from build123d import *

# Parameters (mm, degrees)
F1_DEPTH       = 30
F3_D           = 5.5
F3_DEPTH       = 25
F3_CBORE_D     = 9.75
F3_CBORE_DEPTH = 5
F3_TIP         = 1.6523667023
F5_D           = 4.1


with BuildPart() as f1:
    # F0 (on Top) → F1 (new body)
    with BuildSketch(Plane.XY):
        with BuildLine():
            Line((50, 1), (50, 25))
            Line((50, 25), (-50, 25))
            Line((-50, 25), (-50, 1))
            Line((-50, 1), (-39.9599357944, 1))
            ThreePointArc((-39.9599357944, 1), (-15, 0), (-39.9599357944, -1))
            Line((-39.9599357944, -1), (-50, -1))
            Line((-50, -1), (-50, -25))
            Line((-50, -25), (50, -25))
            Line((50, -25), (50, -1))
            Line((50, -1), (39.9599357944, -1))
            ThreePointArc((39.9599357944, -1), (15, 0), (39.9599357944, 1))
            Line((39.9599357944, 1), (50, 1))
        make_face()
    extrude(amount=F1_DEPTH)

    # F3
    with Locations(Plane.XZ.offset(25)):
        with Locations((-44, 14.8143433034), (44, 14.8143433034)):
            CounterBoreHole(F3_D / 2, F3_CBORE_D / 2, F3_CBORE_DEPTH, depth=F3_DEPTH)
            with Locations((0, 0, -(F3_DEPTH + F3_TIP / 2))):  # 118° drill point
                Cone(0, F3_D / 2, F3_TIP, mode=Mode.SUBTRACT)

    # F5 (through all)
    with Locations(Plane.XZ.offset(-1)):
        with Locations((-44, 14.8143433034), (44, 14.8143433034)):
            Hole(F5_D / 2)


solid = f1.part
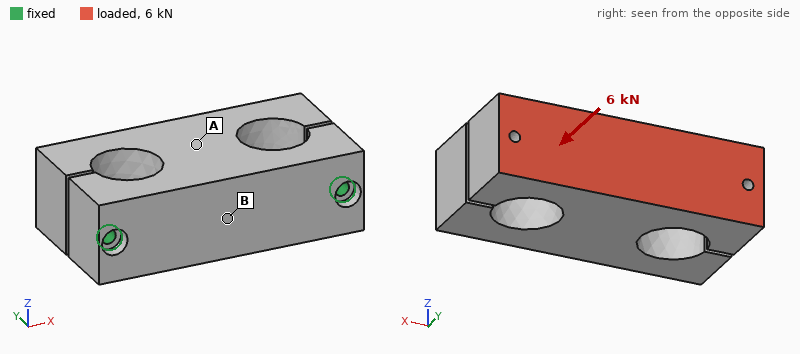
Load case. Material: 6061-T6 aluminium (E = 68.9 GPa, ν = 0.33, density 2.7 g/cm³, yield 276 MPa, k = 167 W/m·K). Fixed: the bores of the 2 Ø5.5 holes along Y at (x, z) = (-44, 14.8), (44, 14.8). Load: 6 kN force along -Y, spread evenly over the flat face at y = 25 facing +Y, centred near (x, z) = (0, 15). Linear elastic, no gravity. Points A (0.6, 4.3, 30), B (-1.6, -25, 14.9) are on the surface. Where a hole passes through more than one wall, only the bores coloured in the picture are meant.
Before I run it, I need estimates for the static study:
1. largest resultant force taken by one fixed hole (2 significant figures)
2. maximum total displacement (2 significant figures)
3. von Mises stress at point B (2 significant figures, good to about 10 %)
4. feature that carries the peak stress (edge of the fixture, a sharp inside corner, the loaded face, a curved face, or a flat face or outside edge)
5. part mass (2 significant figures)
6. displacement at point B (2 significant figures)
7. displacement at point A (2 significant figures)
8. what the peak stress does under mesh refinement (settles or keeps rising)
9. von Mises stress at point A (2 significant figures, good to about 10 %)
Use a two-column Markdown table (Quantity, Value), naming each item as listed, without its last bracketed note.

| Quantity | Value |
|---|---|
| largest resultant force taken by one fixed hole | 3.1 kN |
| maximum total displacement | 73 µm |
| von Mises stress at point B | 24 MPa |
| feature that carries the peak stress | edge of the fixture |
| part mass | 320 g |
| displacement at point B | 30 µm |
| displacement at point A | 31 µm |
| what the peak stress does under mesh refinement | keeps rising |
| von Mises stress at point A | 11 MPa |
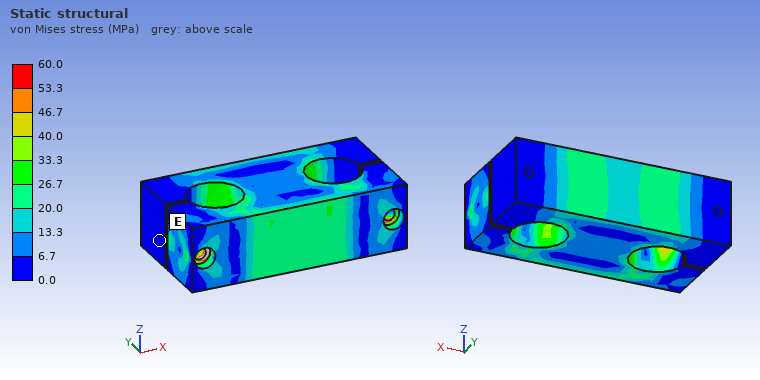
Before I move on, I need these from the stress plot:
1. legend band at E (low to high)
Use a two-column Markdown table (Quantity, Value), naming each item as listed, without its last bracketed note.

| Quantity | Value |
|---|---|
| legend band at E | 0.0 to 6.7 MPa |
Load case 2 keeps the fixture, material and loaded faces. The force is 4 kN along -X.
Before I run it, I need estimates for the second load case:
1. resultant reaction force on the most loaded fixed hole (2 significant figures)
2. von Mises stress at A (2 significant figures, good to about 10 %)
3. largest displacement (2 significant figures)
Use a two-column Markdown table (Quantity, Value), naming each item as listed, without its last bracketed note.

| Quantity | Value |
|---|---|
| resultant reaction force on the most loaded fixed hole | 3.2 kN |
| von Mises stress at A | 14 MPa |
| largest displacement | 98 µm |
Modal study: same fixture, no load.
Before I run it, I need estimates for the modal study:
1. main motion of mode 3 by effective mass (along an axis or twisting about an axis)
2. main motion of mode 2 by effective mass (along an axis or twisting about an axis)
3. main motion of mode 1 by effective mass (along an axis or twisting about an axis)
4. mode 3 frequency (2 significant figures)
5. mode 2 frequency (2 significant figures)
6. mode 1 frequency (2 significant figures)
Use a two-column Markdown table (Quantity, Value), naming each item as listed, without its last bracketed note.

| Quantity | Value |
|---|---|
| main motion of mode 3 by effective mass | twisting about Y |
| main motion of mode 2 by effective mass | along X |
| main motion of mode 1 by effective mass | along Z |
| mode 3 frequency | 3900 Hz |
| mode 2 frequency | 3100 Hz |
| mode 1 frequency | 1900 Hz |
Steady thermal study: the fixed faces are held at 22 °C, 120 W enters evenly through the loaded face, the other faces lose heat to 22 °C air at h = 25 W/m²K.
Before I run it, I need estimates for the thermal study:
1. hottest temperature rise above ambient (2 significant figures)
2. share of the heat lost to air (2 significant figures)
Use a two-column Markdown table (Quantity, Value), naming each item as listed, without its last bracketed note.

| Quantity | Value |
|---|---|
| hottest temperature rise above ambient | 57 K |
| share of the heat lost to air | 13 % |
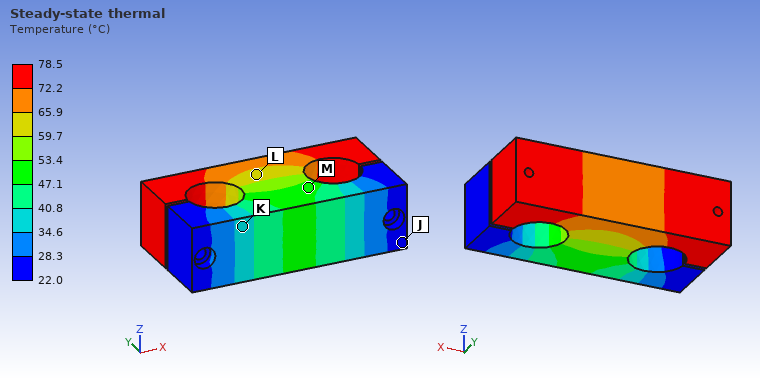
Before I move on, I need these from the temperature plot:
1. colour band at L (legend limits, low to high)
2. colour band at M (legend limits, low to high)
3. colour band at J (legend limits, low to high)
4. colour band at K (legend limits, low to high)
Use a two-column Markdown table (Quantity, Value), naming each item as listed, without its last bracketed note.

| Quantity | Value |
|---|---|
| colour band at L | 59.7 to 65.9 °C |
| colour band at M | 47.1 to 53.4 °C |
| colour band at J | 22.0 to 28.3 °C |
| colour band at K | 34.6 to 40.8 °C |
